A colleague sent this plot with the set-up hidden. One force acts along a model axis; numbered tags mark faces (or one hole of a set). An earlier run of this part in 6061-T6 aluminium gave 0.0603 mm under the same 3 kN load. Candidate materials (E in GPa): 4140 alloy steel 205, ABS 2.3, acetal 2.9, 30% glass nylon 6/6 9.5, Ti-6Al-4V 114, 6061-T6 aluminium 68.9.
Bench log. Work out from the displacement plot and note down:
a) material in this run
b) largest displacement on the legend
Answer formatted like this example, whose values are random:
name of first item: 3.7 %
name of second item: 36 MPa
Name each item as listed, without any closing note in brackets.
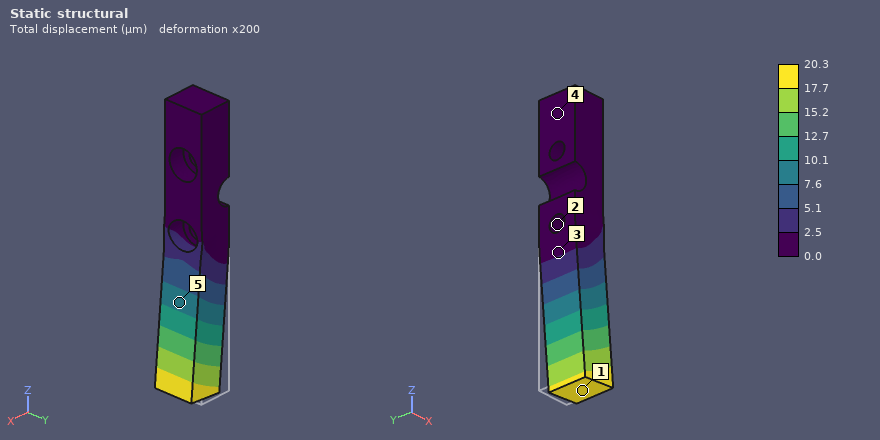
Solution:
material in this run: 4140 alloy steel
largest displacement on the legend: 20.3 µm
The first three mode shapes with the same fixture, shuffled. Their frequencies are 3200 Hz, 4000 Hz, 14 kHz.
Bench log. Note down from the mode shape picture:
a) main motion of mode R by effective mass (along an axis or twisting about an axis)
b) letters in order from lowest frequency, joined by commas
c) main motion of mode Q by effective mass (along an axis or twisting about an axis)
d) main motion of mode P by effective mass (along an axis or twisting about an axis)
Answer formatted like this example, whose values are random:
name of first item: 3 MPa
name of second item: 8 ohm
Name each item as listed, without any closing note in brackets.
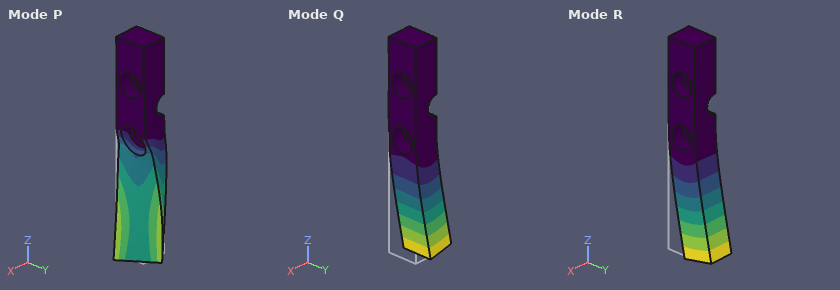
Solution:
main motion of mode R by effective mass: along Y
letters in order from lowest frequency, joined by commas: Q, R, P
main motion of mode Q by effective mass: along X
main motion of mode P by effective mass: twisting about Z
